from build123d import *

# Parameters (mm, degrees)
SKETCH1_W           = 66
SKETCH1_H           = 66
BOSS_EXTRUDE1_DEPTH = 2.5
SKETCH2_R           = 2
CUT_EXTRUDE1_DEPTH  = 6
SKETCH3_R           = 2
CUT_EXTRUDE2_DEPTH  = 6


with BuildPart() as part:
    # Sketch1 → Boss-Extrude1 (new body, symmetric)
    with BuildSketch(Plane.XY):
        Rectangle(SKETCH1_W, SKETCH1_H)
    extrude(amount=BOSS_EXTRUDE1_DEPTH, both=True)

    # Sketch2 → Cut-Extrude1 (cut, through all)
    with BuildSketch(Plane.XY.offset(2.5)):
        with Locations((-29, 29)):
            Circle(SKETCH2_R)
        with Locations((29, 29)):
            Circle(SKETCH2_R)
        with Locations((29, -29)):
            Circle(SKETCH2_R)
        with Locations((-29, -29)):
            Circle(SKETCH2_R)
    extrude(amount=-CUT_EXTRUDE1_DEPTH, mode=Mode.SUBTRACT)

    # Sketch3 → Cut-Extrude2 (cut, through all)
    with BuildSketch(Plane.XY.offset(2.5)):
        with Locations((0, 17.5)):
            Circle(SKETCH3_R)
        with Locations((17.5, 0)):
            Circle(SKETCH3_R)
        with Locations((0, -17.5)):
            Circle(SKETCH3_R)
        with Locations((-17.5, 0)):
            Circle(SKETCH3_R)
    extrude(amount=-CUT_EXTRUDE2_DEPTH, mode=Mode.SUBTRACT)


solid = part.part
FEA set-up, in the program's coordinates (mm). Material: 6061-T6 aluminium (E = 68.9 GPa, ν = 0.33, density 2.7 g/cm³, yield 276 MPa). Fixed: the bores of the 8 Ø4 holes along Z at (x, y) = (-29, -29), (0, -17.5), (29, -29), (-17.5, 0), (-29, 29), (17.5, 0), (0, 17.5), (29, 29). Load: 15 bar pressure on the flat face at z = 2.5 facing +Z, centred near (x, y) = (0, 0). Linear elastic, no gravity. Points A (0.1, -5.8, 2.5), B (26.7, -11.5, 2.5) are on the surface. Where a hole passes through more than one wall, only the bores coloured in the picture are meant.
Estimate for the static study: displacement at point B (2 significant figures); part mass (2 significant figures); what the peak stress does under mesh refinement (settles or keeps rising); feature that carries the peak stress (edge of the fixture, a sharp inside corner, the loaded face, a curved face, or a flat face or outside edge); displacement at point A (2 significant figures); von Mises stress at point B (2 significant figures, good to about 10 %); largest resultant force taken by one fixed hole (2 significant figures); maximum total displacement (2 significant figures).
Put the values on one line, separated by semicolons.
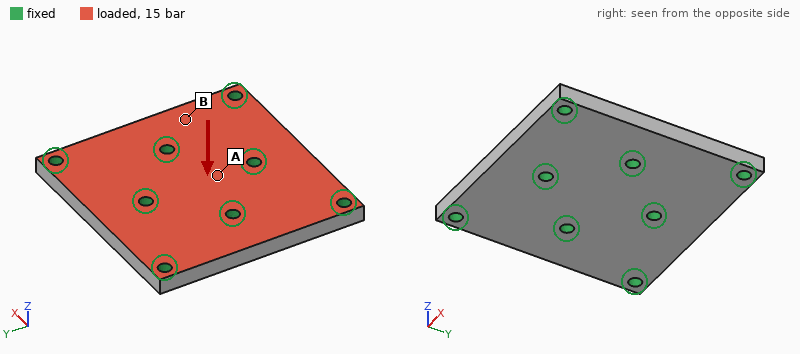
8.2 µm; 57 g; keeps rising; edge of the fixture; 3.2 µm; 15 MPa; 1.1 kN; 13 µm
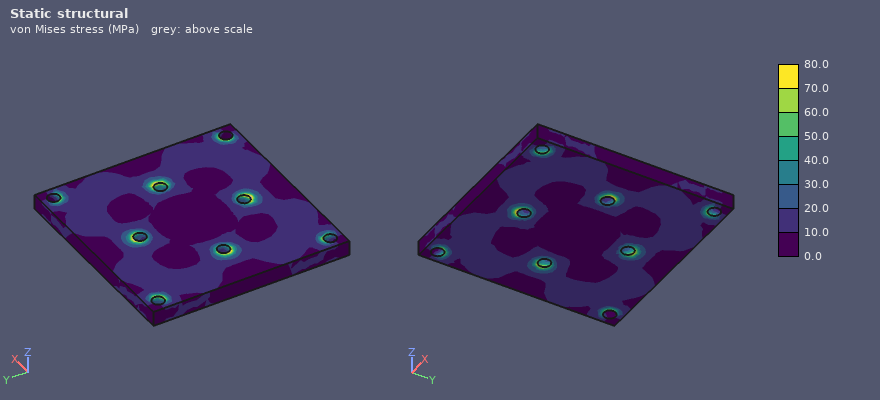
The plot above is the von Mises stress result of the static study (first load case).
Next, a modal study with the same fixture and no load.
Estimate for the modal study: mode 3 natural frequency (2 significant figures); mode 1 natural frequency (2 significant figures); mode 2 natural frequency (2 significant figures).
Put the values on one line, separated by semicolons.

18 kHz; 17 kHz; 18 kHz
